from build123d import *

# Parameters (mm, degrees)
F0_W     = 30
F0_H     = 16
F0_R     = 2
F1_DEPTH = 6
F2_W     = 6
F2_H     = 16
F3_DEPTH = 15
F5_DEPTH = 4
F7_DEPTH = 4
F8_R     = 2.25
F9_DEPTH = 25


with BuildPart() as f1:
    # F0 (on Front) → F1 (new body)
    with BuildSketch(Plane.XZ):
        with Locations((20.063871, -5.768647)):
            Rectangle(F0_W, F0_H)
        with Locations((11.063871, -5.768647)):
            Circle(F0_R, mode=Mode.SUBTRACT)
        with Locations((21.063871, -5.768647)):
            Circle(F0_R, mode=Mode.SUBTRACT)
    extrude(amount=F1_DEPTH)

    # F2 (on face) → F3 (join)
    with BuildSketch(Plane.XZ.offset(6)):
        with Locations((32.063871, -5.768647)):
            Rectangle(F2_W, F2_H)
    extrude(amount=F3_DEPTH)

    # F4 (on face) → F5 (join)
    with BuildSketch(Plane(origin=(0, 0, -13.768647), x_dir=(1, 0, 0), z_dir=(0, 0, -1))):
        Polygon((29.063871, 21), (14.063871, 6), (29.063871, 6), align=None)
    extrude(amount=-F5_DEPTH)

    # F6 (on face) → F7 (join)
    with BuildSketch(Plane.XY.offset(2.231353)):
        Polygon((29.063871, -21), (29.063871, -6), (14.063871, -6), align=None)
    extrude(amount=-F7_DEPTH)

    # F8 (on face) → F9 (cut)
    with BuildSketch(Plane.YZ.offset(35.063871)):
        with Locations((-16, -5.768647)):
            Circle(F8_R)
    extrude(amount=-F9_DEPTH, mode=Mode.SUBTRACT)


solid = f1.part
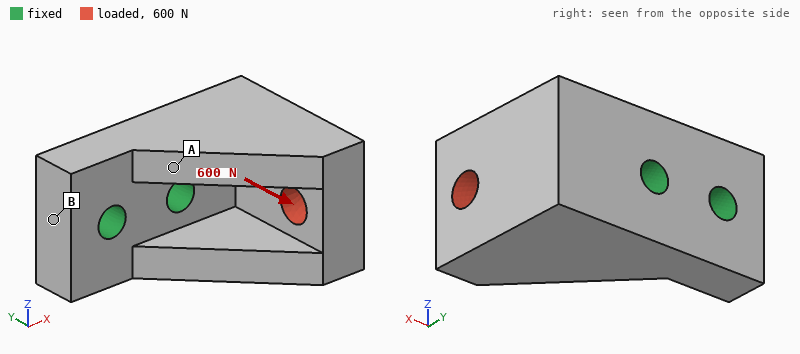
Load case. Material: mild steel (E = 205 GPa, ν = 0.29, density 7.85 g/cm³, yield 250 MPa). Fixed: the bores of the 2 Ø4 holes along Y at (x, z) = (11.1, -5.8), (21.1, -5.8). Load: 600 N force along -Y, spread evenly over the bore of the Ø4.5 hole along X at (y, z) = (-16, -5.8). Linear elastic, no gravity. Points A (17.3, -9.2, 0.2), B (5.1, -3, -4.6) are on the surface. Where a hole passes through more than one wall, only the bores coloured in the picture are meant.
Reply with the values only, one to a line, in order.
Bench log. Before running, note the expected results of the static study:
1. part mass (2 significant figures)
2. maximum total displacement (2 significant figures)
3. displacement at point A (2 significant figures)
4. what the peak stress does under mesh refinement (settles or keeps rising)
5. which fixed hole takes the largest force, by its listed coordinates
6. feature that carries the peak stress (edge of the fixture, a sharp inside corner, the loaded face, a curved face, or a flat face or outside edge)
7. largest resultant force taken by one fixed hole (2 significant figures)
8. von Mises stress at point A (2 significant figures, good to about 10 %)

39 g
6.3 µm
1.0 µm
keeps rising
(21.1, -5.8)
edge of the fixture
860 N
19 MPa
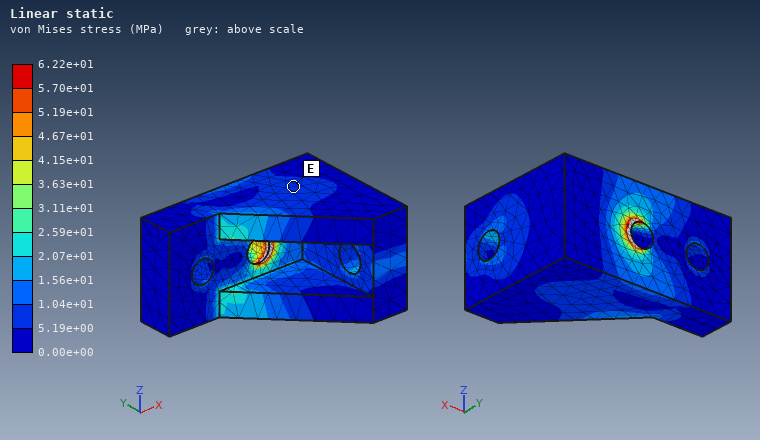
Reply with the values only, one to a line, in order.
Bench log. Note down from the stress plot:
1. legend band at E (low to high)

5.19e+00 to 1.04e+01 MPa
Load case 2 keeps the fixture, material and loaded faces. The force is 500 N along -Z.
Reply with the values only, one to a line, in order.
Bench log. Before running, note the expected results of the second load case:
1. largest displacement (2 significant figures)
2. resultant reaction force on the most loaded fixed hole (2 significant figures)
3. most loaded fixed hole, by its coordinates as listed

10 µm
810 N
(21.1, -5.8)
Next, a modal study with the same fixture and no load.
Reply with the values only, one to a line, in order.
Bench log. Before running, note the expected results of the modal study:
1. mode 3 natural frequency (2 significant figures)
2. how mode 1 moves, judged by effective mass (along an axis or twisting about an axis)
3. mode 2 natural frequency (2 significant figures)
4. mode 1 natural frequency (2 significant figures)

23 kHz
along Z
13 kHz
12 kHz
